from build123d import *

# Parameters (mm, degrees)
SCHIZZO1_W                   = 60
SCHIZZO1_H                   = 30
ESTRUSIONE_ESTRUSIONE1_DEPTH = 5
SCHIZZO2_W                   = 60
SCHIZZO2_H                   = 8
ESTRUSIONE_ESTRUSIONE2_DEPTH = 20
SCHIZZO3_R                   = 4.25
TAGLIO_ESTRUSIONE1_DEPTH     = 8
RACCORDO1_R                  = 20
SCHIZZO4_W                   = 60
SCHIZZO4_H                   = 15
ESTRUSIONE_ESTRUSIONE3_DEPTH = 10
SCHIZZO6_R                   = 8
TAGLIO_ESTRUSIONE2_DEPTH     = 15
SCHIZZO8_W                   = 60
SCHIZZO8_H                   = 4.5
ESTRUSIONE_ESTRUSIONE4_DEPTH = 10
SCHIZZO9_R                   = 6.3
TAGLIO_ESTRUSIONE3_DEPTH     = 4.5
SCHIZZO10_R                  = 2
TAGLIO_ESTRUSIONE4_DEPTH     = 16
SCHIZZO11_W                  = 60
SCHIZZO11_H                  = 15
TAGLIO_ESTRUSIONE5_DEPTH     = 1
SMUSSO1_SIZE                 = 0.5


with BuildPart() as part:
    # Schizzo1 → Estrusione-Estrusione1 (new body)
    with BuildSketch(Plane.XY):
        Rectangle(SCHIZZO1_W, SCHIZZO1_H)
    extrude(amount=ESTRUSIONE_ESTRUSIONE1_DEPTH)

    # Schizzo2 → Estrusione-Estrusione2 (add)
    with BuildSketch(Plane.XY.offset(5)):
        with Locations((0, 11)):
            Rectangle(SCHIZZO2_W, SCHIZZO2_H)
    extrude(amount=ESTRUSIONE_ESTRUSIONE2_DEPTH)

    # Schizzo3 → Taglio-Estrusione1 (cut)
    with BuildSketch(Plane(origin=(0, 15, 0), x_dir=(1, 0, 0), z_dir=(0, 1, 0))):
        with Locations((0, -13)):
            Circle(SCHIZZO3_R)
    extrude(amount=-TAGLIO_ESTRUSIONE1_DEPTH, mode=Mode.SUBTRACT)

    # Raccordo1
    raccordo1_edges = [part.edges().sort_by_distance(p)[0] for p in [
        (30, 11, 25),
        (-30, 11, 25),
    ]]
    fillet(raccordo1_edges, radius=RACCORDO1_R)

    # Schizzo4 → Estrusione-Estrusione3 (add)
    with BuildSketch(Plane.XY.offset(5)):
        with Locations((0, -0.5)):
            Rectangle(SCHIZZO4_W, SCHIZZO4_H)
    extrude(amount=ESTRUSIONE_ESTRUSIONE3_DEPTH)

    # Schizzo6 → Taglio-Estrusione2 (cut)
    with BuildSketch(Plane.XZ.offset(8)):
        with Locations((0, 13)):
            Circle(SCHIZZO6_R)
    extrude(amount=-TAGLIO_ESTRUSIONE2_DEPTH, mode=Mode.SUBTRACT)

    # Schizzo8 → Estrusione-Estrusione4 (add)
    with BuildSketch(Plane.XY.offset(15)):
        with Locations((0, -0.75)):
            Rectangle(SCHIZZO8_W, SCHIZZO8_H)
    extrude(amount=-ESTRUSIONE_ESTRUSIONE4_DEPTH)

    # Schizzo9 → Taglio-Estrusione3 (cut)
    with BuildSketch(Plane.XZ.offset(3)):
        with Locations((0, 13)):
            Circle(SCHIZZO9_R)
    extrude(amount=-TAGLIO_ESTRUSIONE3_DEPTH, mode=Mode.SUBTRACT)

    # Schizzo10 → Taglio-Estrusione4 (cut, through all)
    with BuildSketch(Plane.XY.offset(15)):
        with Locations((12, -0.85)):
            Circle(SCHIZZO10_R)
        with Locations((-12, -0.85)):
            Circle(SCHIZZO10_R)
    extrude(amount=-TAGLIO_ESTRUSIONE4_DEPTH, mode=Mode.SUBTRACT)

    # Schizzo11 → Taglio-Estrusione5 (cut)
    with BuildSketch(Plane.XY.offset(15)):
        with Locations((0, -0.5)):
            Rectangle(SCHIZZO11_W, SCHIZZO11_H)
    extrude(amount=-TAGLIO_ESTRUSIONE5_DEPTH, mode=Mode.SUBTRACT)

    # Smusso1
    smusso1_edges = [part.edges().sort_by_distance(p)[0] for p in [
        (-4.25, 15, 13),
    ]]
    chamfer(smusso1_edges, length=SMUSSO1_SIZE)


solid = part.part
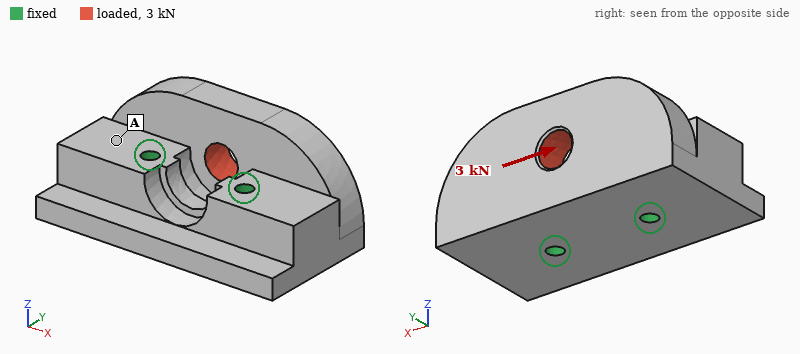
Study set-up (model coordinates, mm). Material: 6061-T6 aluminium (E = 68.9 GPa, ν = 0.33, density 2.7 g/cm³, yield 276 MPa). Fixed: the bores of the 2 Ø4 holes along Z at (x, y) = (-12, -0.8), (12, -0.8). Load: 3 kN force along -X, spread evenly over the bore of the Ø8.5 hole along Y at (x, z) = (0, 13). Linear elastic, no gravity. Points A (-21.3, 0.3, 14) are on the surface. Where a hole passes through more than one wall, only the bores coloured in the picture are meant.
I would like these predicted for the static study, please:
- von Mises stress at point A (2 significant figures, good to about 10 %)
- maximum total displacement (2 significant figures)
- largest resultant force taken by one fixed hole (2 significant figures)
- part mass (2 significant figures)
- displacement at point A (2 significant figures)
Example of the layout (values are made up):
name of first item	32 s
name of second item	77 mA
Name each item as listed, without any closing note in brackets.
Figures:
von Mises stress at point A	6.3 MPa
maximum total displacement	9.7 µm
largest resultant force taken by one fixed hole	1.9 kN
part mass	62 g
displacement at point A	2.8 µm
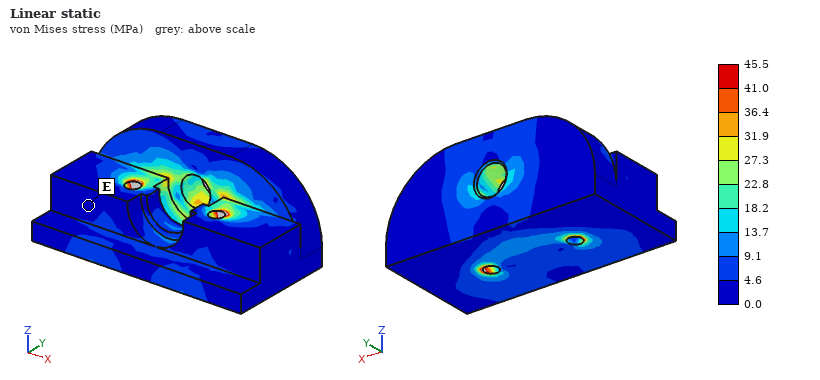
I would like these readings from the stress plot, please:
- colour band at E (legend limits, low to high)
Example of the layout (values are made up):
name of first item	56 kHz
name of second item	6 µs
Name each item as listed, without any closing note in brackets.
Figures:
colour band at E	0.0 to 4.6 MPa
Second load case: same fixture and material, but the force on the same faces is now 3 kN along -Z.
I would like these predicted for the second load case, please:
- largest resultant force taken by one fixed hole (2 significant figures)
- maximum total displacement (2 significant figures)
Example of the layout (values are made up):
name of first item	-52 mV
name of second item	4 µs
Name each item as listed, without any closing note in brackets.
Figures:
largest resultant force taken by one fixed hole	1.5 kN
maximum total displacement	16 µm
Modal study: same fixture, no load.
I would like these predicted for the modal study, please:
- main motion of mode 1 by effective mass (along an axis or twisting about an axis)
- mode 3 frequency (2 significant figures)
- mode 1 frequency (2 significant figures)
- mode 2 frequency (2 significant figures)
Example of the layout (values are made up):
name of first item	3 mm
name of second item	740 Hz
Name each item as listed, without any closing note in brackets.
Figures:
main motion of mode 1 by effective mass	along Z
mode 3 frequency	18 kHz
mode 1 frequency	15 kHz
mode 2 frequency	15 kHz
